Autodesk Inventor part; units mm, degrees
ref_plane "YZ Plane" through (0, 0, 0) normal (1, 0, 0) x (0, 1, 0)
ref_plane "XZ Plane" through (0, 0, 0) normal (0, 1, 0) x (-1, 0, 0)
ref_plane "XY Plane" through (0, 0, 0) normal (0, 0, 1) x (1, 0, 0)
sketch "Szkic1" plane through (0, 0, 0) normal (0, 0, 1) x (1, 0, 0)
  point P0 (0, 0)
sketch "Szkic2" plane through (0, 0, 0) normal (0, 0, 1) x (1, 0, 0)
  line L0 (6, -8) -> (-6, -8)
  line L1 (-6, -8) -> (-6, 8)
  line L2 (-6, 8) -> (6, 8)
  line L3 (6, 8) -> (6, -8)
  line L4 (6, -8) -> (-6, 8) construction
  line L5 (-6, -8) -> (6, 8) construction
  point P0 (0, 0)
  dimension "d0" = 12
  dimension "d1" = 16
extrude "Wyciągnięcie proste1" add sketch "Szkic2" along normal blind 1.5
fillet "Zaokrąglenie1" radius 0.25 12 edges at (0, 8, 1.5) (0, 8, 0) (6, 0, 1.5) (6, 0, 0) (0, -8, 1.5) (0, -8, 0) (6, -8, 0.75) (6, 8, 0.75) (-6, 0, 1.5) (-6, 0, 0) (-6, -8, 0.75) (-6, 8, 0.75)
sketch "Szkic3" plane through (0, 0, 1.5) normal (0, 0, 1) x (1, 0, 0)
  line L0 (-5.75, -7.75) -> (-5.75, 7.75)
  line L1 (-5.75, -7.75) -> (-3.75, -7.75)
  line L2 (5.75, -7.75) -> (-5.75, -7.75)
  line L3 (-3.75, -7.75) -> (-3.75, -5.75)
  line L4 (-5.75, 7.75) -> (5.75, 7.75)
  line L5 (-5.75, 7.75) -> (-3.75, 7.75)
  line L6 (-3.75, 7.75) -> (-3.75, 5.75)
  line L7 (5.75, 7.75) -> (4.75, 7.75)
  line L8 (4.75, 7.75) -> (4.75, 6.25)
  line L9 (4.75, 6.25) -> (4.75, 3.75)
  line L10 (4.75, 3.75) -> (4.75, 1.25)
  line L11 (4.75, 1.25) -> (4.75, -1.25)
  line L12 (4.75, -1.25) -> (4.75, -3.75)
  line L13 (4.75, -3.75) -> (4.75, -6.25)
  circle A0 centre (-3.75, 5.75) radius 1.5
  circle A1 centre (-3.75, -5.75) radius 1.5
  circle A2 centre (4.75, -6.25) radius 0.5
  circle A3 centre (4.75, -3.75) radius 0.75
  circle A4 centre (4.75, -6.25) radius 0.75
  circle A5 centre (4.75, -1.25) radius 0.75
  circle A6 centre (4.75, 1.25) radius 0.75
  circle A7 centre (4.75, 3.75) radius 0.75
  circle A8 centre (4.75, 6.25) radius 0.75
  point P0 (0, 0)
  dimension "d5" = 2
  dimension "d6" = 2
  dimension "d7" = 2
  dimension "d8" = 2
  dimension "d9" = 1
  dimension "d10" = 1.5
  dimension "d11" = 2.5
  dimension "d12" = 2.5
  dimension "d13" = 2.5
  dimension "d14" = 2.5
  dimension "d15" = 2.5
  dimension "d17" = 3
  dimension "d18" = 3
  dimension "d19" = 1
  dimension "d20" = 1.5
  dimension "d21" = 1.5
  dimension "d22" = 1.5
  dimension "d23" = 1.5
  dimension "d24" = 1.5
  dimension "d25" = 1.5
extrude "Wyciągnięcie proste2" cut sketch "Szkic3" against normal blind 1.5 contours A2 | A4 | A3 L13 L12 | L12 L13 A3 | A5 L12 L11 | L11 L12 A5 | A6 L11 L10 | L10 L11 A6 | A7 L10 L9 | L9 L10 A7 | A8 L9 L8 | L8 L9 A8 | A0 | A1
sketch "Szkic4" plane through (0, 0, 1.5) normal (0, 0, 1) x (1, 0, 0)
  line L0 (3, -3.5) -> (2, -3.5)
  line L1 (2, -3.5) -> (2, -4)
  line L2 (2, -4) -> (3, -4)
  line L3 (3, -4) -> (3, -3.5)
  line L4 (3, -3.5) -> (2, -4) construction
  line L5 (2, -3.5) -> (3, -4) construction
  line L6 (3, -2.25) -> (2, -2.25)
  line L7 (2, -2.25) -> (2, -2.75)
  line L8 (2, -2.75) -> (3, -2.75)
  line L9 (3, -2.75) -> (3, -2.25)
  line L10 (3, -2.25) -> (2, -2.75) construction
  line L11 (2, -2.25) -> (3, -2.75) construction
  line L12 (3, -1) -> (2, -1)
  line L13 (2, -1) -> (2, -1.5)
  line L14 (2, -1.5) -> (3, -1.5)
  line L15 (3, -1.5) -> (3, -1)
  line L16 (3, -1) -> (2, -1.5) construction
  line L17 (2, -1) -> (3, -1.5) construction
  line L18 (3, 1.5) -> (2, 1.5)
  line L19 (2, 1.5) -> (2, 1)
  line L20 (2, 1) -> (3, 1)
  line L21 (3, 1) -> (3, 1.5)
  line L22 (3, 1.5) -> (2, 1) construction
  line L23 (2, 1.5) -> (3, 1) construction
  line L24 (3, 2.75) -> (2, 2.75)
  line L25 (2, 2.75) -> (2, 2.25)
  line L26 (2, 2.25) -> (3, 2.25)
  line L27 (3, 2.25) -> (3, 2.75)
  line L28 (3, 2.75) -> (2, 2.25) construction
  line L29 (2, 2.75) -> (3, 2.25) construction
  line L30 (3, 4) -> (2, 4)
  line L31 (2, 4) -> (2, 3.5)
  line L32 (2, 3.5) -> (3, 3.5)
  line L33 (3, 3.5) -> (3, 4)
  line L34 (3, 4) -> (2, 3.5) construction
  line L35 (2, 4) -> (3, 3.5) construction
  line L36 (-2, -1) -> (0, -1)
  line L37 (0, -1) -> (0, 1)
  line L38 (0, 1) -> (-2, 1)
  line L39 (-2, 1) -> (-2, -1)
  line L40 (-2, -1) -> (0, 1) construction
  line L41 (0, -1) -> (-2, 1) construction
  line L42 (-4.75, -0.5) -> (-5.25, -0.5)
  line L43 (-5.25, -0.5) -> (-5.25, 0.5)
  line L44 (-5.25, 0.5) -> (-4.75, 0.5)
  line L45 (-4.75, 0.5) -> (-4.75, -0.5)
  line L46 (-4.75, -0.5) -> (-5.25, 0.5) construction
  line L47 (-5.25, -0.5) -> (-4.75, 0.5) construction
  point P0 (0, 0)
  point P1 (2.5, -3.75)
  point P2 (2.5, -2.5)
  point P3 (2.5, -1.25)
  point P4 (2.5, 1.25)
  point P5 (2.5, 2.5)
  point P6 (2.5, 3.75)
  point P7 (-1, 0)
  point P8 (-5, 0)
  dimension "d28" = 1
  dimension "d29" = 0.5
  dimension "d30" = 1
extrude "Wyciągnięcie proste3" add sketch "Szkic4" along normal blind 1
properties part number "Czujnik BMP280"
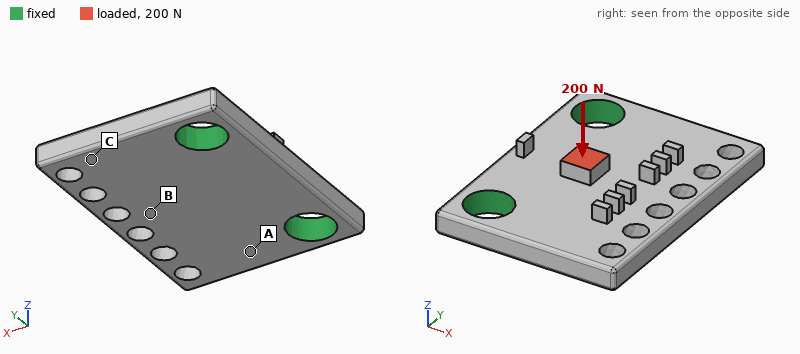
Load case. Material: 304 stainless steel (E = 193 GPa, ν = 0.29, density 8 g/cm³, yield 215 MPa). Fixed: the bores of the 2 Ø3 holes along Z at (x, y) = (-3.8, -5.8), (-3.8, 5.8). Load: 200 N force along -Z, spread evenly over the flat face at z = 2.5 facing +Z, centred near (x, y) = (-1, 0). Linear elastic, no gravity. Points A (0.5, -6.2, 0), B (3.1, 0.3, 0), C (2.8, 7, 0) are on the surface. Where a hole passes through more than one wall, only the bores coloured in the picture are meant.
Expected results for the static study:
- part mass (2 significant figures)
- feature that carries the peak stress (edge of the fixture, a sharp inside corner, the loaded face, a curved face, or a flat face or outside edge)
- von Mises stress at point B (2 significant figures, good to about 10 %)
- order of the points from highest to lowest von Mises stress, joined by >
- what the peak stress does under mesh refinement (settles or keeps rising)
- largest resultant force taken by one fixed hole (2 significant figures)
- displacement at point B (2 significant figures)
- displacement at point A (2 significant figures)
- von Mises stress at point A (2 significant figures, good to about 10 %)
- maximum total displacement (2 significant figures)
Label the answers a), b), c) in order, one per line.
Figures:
a) 2.1 g
b) edge of the fixture
c) 40 MPa
d) B > A > C
e) keeps rising
f) 100 N
g) 7.3 µm
h) 1.7 µm
i) 26 MPa
j) 9.7 µm
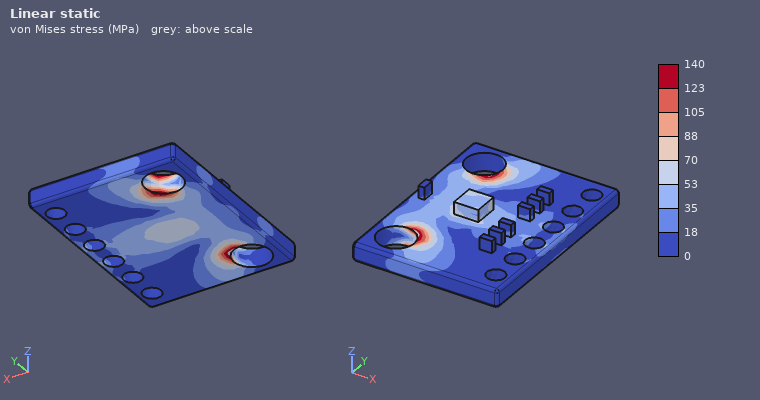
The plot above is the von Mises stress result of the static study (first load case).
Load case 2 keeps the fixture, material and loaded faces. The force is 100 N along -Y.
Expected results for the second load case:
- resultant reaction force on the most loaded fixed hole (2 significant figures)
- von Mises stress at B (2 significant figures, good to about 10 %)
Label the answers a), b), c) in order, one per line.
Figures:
a) 58 N
b) 3.5 MPa
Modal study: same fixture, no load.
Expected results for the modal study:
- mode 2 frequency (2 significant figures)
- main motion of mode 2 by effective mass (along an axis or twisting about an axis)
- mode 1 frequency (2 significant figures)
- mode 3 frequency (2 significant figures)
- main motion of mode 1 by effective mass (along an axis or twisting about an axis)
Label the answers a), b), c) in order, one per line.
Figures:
a) 26 kHz
b) twisting about X
c) 16 kHz
d) 43 kHz
e) along Z
